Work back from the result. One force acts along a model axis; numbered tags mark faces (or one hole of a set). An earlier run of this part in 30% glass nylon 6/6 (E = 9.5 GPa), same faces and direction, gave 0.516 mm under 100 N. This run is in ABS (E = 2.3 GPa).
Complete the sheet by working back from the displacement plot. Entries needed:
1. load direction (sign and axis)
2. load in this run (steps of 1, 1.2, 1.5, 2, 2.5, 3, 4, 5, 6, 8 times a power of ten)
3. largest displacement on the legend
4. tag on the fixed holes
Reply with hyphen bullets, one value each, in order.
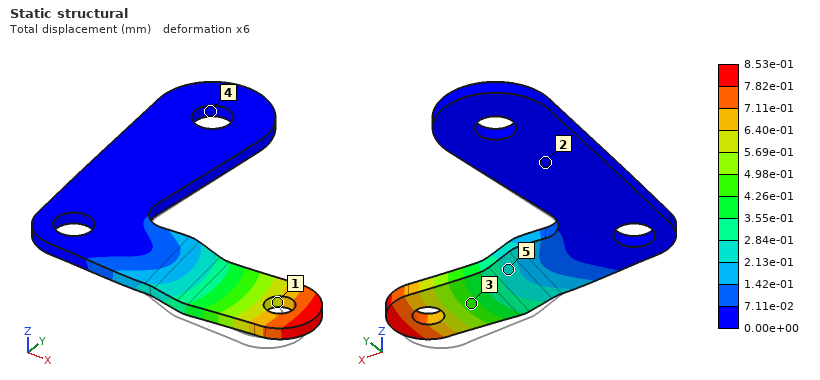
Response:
- +Y
- 40 N
- 8.53e-01 mm
- 4
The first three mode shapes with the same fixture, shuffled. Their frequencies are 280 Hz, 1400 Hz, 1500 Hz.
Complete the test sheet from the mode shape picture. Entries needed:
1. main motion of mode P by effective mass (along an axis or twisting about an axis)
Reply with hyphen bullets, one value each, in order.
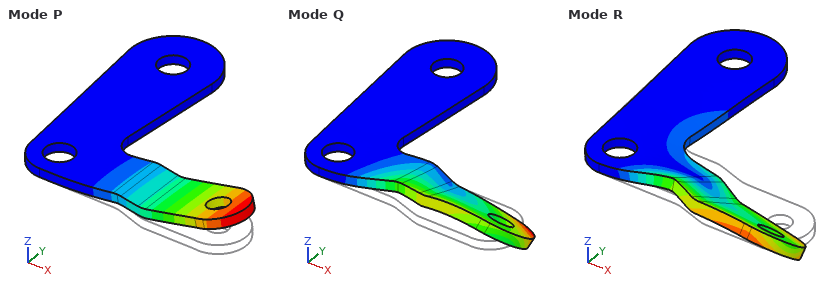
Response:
- along Z
